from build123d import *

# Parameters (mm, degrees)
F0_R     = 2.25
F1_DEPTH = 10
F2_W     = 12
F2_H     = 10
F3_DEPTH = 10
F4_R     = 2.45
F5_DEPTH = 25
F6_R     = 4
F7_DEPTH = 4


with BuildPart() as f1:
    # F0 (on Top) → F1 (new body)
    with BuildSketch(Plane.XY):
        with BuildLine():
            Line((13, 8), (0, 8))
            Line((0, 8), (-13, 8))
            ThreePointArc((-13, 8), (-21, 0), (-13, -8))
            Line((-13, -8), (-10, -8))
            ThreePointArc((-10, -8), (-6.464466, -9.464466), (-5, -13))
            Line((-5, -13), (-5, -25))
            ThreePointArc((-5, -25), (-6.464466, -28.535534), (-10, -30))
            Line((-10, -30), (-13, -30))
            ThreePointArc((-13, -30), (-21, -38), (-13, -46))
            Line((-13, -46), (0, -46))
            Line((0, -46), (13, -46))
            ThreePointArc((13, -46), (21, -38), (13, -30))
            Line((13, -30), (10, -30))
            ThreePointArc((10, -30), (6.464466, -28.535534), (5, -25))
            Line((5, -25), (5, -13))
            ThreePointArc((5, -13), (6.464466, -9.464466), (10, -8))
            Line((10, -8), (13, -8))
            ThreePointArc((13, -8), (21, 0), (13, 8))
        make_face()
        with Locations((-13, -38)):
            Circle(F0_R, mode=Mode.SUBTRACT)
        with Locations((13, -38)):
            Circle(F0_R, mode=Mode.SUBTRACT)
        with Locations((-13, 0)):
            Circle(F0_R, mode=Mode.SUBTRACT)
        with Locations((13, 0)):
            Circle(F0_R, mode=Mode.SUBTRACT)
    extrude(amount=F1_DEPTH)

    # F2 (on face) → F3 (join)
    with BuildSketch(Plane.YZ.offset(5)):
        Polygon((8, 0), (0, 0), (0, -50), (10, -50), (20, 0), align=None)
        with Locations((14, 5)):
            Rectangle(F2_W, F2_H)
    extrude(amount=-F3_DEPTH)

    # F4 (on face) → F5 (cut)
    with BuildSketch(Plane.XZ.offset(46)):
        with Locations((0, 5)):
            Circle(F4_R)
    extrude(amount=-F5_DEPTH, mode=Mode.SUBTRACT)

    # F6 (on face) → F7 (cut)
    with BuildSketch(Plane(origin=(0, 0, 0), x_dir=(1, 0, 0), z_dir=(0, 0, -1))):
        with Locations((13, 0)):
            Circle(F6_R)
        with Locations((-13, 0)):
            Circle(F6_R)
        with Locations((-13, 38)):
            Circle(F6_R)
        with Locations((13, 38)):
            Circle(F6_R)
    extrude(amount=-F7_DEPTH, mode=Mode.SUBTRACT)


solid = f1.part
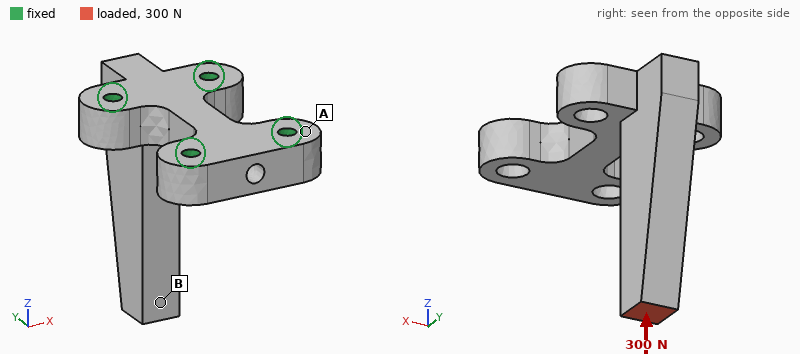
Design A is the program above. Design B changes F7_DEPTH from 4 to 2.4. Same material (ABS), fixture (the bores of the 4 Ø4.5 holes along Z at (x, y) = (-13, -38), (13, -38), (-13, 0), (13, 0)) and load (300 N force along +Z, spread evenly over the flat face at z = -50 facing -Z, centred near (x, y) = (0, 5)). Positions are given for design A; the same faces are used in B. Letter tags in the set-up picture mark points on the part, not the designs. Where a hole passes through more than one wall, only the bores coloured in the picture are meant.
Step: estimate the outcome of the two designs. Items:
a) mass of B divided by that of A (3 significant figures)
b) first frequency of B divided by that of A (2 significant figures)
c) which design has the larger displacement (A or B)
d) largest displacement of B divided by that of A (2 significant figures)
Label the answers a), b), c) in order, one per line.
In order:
a) 1.01
b) 1.0
c) A
d) 0.86
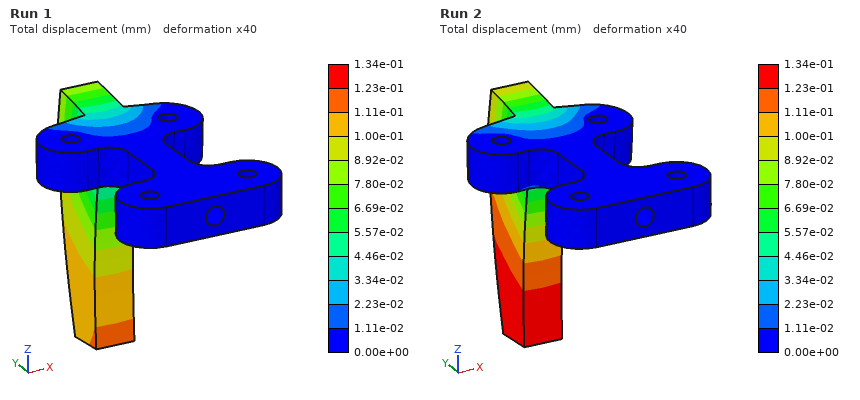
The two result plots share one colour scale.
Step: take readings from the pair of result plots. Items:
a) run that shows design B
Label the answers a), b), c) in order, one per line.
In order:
a) Run 1
